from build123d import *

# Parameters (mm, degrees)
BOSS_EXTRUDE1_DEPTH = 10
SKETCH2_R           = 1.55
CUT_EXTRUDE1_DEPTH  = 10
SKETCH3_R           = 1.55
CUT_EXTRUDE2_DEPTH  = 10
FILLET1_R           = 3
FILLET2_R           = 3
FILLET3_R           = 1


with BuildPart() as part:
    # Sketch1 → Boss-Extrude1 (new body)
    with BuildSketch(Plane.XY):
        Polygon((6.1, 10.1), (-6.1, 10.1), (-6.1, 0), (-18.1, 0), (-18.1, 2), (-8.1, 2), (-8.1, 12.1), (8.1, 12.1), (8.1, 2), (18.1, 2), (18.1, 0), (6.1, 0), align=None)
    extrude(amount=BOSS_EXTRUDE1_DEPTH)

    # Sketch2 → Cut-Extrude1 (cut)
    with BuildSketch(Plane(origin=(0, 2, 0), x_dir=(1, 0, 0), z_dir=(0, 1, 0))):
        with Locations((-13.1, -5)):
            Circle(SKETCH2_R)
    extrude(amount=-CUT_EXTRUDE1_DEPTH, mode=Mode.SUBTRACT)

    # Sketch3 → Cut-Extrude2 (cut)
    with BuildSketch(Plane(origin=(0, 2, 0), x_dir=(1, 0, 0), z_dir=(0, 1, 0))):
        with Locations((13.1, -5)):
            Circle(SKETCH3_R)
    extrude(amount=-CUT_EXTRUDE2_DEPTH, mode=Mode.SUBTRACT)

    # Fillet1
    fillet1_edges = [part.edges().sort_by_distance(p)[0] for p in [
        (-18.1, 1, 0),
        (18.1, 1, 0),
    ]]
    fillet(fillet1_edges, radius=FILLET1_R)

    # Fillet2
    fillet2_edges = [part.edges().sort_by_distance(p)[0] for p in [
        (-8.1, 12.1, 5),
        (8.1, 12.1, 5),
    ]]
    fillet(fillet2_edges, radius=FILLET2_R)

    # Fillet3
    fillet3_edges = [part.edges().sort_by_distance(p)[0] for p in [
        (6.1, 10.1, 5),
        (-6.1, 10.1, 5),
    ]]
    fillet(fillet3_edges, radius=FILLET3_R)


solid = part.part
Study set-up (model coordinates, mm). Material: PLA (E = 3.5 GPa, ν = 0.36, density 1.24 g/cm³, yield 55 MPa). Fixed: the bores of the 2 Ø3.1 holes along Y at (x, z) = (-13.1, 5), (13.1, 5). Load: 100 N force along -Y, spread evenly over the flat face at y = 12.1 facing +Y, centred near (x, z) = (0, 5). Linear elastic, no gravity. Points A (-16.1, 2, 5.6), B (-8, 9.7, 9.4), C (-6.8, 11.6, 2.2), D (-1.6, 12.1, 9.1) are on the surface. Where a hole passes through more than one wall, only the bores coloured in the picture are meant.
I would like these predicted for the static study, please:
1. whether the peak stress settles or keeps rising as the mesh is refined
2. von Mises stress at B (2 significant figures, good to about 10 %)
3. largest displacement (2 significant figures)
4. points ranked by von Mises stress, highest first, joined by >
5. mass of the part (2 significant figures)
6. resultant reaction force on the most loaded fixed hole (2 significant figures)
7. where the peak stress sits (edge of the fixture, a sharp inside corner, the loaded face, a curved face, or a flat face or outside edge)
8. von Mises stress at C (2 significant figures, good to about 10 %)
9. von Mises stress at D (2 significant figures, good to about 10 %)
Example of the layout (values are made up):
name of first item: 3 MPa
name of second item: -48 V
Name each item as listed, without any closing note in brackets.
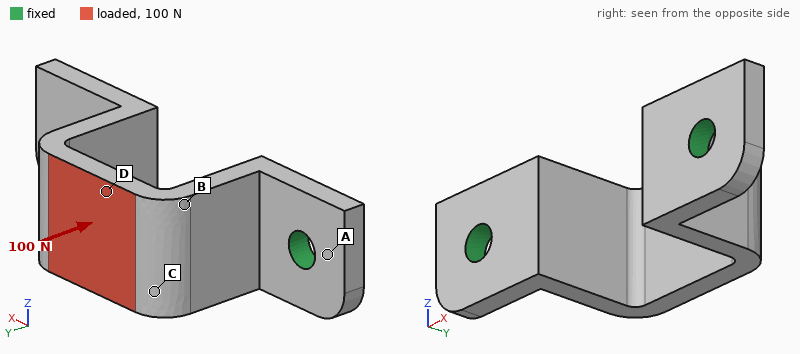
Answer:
whether the peak stress settles or keeps rising as the mesh is refined: keeps rising
von Mises stress at B: 8.0 MPa
largest displacement: 0.12 mm
points ranked by von Mises stress, highest first, joined by >: D > B > C > A
mass of the part: 1.3 g
resultant reaction force on the most loaded fixed hole: 56 N
where the peak stress sits: edge of the fixture
von Mises stress at C: 6.0 MPa
von Mises stress at D: 13 MPa
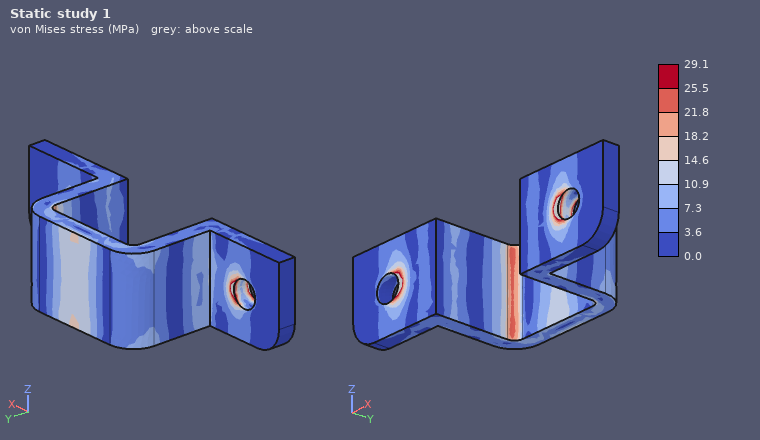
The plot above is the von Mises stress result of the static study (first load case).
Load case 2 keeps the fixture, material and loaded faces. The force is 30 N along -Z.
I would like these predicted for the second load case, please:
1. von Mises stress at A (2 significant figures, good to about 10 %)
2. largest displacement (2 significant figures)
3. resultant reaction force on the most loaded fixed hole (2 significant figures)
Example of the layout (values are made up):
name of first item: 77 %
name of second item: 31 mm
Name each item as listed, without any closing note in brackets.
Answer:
von Mises stress at A: 3.2 MPa
largest displacement: 0.25 mm
resultant reaction force on the most loaded fixed hole: 15 N
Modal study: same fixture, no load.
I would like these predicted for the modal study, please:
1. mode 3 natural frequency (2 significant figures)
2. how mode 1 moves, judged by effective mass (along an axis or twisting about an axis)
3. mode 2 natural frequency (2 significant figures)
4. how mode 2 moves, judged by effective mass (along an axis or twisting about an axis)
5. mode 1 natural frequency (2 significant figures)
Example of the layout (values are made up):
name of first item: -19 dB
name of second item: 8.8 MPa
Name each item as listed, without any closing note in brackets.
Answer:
mode 3 natural frequency: 5300 Hz
how mode 1 moves, judged by effective mass: along Z
mode 2 natural frequency: 3800 Hz
how mode 2 moves, judged by effective mass: along X
mode 1 natural frequency: 2700 Hz
